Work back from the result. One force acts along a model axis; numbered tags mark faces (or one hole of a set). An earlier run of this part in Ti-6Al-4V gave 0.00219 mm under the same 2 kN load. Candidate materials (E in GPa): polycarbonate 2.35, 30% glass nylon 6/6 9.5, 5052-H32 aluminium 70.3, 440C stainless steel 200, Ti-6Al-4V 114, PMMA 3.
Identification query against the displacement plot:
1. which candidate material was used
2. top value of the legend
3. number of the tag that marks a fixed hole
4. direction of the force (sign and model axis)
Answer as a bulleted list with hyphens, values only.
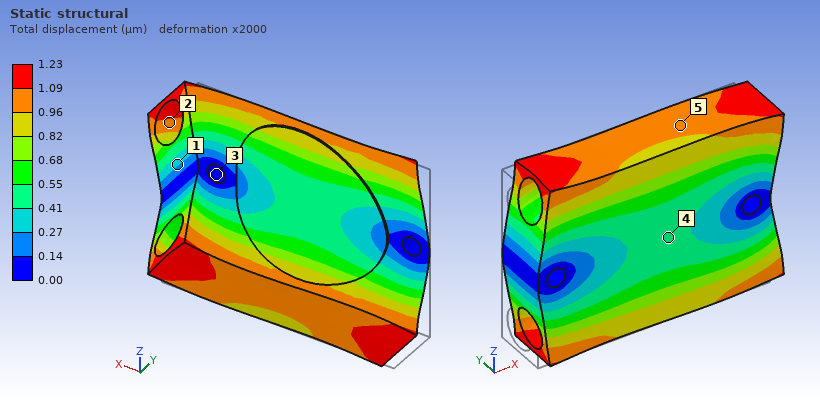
- 440C stainless steel
- 1.23 µm
- 3
- +X
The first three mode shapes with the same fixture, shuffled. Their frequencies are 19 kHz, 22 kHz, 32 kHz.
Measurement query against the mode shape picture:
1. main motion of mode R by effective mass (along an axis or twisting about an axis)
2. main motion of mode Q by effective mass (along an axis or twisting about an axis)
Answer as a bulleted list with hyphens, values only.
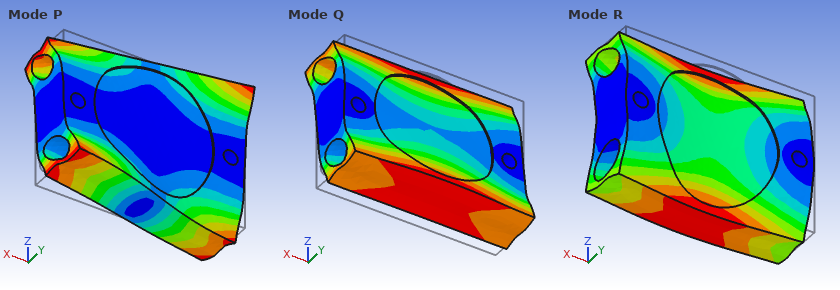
- along Y
- twisting about X
